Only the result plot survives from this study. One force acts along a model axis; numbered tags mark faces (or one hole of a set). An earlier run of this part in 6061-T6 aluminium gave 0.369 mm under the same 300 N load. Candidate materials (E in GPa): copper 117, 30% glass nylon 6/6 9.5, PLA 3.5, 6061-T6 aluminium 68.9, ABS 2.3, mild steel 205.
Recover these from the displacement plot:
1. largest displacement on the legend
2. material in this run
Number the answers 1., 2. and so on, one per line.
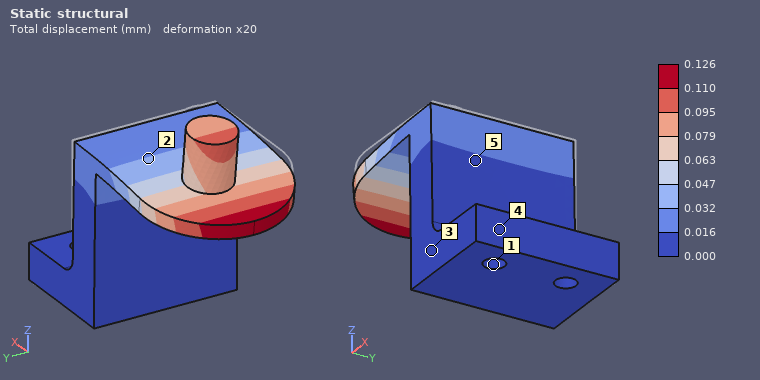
1. 0.126 mm
2. mild steel
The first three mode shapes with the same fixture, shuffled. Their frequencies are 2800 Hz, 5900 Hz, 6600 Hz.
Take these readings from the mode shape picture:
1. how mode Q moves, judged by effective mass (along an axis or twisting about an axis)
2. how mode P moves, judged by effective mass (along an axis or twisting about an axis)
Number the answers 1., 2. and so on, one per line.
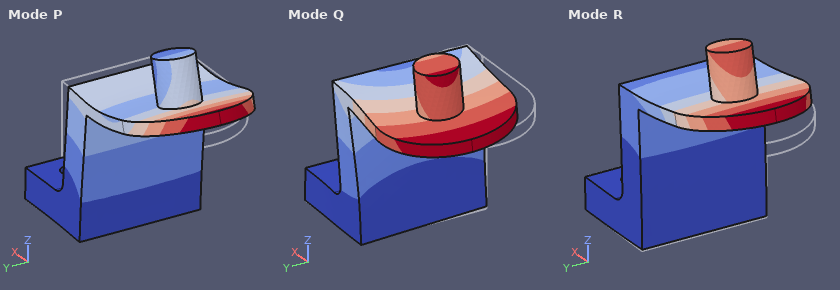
1. along Y
2. along X
